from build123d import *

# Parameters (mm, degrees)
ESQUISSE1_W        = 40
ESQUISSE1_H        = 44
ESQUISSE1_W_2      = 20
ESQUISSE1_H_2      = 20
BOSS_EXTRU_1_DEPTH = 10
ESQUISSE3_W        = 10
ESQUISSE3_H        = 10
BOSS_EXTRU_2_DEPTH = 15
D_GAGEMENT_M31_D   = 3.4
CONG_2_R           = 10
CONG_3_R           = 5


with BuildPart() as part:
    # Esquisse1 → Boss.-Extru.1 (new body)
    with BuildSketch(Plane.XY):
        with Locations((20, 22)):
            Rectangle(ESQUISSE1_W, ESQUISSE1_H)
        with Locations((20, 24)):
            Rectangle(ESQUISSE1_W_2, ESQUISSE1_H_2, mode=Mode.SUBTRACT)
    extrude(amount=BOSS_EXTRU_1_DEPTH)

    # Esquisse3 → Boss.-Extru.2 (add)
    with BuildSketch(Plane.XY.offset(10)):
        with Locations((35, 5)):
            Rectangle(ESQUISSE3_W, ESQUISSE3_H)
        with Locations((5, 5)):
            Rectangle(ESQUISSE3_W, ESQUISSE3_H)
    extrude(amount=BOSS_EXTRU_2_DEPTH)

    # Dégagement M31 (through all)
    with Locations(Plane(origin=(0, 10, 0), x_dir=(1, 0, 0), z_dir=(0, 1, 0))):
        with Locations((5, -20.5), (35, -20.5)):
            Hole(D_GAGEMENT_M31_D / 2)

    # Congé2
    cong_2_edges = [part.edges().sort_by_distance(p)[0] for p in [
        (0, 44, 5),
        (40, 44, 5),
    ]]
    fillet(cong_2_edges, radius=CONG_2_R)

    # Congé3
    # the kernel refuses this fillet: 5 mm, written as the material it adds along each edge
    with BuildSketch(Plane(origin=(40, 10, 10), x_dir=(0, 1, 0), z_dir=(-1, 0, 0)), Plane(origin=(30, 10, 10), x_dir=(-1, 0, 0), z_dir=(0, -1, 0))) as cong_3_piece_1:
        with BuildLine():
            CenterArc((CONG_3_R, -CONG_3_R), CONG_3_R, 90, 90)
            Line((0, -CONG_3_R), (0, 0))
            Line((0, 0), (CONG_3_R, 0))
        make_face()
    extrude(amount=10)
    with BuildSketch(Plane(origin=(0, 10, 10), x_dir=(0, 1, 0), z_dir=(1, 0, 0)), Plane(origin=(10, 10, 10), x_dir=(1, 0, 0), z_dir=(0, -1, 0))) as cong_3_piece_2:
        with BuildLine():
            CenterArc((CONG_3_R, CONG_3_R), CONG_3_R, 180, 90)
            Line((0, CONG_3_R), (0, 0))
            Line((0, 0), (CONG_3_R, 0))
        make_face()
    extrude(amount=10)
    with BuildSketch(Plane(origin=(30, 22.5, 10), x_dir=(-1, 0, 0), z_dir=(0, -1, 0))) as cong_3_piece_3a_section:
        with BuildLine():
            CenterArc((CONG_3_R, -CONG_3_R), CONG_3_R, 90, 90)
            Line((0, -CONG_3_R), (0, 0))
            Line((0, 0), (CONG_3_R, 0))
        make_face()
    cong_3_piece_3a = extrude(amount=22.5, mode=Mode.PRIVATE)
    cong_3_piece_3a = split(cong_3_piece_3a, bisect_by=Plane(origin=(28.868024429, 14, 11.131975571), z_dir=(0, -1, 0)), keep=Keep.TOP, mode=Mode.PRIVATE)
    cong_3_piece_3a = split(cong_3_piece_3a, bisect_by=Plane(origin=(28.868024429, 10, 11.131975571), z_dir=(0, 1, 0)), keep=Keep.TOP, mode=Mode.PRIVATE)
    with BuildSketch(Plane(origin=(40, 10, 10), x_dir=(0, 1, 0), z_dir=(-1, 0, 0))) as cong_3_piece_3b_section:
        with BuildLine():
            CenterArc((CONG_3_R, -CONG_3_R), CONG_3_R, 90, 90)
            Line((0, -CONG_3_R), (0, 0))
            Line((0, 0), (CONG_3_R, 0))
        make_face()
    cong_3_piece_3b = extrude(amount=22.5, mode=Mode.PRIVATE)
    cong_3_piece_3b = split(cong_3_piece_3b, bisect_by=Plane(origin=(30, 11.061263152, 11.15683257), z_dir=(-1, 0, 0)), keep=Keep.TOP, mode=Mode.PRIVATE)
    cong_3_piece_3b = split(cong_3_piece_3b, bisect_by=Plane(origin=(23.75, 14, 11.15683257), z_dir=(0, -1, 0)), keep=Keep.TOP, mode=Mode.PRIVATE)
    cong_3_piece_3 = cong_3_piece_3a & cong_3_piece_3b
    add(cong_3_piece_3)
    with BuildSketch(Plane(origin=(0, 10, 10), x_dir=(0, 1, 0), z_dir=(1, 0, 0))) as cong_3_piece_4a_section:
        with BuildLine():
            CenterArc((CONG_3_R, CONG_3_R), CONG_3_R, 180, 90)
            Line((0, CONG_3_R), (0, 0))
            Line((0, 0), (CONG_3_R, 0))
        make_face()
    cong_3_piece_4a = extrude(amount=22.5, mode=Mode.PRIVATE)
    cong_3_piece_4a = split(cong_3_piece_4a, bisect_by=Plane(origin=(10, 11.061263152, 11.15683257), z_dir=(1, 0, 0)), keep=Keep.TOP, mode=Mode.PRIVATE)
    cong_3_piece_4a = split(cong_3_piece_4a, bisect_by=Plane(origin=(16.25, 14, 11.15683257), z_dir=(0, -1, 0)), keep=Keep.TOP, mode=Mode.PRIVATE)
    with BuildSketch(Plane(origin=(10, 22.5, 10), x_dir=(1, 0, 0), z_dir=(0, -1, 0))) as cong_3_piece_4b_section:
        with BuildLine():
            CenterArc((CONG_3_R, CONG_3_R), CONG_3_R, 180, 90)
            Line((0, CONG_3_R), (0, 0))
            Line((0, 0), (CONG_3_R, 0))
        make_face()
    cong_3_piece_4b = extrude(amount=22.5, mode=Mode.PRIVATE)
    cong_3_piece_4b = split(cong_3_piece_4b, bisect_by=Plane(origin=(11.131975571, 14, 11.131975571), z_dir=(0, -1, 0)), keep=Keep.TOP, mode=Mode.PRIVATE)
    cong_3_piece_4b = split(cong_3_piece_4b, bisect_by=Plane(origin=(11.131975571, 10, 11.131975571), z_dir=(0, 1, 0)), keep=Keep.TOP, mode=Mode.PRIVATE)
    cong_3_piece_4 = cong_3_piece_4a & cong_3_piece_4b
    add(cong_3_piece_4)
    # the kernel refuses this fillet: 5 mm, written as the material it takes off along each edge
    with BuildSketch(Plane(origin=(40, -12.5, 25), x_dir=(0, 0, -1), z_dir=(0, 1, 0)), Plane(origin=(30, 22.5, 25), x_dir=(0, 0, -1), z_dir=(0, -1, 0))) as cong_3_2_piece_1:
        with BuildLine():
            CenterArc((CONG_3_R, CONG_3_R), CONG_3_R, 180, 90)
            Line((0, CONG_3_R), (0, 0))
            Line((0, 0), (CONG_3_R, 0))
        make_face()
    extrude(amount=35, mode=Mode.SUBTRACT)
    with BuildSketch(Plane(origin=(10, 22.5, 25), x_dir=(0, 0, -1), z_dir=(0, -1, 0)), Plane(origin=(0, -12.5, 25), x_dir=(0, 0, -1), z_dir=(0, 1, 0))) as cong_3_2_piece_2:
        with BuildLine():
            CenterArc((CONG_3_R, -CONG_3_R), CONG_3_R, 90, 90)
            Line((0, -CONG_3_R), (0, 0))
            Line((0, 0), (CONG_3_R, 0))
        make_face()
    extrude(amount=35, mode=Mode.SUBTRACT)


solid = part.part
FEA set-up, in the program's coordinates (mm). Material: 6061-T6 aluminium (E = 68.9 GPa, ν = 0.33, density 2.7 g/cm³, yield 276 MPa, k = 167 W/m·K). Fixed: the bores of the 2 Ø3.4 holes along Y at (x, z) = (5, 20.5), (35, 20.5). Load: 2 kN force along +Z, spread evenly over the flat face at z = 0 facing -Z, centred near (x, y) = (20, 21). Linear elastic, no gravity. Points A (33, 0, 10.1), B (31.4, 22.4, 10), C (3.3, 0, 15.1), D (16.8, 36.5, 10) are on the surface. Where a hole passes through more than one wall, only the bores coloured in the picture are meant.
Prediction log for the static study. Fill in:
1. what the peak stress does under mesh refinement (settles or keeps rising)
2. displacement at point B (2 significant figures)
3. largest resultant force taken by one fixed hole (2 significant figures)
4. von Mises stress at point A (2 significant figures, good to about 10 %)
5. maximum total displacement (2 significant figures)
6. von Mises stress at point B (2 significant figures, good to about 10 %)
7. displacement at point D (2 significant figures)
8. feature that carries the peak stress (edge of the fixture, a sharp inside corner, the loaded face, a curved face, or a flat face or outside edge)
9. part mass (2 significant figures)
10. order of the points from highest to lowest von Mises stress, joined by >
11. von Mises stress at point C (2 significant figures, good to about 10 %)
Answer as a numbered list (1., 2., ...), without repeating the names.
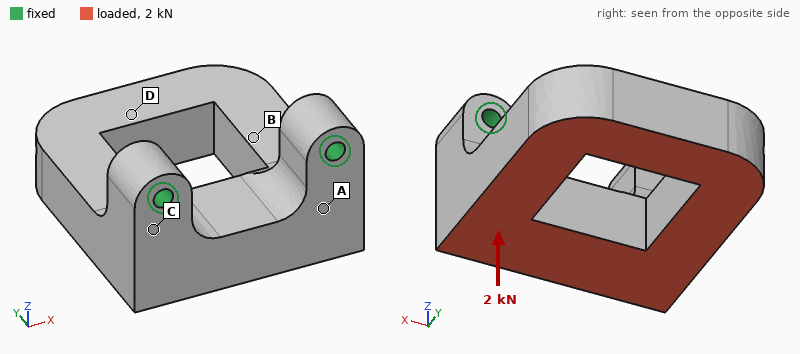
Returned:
1. keeps rising
2. 0.071 mm
3. 1.0 kN
4. 47 MPa
5. 0.20 mm
6. 33 MPa
7. 0.15 mm
8. edge of the fixture
9. 43 g
10. C > A > B > D
11. 82 MPa
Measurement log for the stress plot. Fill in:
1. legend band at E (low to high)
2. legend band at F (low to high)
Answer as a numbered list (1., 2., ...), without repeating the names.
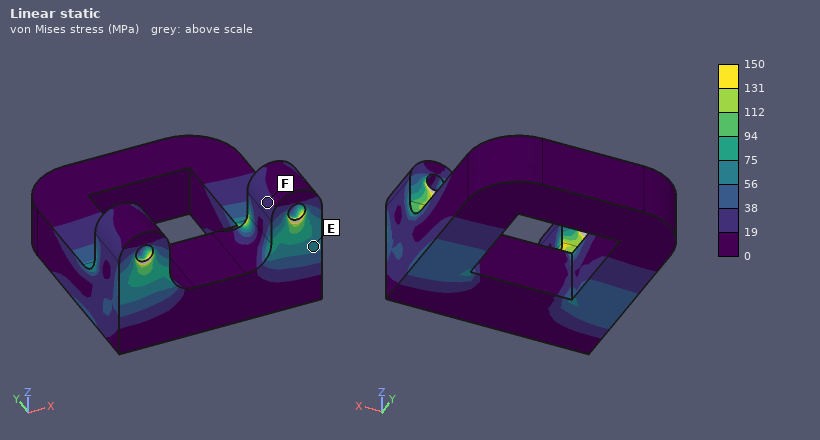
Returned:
1. 56 to 75 MPa
2. 19 to 38 MPa
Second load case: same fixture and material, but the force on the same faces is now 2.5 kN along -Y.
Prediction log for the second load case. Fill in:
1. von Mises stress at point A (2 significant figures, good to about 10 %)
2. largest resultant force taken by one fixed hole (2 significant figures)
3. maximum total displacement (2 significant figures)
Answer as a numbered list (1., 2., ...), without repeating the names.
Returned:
1. 51 MPa
2. 1.3 kN
3. 0.20 mm
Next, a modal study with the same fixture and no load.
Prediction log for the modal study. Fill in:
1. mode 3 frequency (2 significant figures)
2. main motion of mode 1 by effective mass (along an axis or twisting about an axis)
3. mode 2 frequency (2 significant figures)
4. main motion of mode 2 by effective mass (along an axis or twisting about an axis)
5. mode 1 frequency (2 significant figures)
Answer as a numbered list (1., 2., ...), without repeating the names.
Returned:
1. 8800 Hz
2. along Z
3. 5100 Hz
4. along X
5. 3100 Hz
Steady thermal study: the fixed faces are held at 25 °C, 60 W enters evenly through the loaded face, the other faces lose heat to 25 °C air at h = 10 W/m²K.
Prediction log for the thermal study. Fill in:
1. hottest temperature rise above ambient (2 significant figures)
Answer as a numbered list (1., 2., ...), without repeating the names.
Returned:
1. 45 K
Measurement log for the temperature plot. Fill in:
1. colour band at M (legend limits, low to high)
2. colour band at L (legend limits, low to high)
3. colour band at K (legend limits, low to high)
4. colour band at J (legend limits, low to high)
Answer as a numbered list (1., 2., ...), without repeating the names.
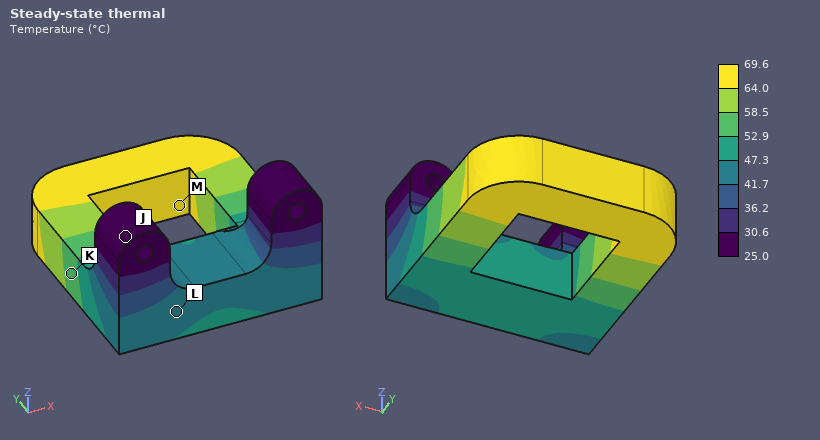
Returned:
1. 64.0 to 69.6 °C
2. 41.7 to 47.3 °C
3. 52.9 to 58.5 °C
4. 25.0 to 30.6 °C
